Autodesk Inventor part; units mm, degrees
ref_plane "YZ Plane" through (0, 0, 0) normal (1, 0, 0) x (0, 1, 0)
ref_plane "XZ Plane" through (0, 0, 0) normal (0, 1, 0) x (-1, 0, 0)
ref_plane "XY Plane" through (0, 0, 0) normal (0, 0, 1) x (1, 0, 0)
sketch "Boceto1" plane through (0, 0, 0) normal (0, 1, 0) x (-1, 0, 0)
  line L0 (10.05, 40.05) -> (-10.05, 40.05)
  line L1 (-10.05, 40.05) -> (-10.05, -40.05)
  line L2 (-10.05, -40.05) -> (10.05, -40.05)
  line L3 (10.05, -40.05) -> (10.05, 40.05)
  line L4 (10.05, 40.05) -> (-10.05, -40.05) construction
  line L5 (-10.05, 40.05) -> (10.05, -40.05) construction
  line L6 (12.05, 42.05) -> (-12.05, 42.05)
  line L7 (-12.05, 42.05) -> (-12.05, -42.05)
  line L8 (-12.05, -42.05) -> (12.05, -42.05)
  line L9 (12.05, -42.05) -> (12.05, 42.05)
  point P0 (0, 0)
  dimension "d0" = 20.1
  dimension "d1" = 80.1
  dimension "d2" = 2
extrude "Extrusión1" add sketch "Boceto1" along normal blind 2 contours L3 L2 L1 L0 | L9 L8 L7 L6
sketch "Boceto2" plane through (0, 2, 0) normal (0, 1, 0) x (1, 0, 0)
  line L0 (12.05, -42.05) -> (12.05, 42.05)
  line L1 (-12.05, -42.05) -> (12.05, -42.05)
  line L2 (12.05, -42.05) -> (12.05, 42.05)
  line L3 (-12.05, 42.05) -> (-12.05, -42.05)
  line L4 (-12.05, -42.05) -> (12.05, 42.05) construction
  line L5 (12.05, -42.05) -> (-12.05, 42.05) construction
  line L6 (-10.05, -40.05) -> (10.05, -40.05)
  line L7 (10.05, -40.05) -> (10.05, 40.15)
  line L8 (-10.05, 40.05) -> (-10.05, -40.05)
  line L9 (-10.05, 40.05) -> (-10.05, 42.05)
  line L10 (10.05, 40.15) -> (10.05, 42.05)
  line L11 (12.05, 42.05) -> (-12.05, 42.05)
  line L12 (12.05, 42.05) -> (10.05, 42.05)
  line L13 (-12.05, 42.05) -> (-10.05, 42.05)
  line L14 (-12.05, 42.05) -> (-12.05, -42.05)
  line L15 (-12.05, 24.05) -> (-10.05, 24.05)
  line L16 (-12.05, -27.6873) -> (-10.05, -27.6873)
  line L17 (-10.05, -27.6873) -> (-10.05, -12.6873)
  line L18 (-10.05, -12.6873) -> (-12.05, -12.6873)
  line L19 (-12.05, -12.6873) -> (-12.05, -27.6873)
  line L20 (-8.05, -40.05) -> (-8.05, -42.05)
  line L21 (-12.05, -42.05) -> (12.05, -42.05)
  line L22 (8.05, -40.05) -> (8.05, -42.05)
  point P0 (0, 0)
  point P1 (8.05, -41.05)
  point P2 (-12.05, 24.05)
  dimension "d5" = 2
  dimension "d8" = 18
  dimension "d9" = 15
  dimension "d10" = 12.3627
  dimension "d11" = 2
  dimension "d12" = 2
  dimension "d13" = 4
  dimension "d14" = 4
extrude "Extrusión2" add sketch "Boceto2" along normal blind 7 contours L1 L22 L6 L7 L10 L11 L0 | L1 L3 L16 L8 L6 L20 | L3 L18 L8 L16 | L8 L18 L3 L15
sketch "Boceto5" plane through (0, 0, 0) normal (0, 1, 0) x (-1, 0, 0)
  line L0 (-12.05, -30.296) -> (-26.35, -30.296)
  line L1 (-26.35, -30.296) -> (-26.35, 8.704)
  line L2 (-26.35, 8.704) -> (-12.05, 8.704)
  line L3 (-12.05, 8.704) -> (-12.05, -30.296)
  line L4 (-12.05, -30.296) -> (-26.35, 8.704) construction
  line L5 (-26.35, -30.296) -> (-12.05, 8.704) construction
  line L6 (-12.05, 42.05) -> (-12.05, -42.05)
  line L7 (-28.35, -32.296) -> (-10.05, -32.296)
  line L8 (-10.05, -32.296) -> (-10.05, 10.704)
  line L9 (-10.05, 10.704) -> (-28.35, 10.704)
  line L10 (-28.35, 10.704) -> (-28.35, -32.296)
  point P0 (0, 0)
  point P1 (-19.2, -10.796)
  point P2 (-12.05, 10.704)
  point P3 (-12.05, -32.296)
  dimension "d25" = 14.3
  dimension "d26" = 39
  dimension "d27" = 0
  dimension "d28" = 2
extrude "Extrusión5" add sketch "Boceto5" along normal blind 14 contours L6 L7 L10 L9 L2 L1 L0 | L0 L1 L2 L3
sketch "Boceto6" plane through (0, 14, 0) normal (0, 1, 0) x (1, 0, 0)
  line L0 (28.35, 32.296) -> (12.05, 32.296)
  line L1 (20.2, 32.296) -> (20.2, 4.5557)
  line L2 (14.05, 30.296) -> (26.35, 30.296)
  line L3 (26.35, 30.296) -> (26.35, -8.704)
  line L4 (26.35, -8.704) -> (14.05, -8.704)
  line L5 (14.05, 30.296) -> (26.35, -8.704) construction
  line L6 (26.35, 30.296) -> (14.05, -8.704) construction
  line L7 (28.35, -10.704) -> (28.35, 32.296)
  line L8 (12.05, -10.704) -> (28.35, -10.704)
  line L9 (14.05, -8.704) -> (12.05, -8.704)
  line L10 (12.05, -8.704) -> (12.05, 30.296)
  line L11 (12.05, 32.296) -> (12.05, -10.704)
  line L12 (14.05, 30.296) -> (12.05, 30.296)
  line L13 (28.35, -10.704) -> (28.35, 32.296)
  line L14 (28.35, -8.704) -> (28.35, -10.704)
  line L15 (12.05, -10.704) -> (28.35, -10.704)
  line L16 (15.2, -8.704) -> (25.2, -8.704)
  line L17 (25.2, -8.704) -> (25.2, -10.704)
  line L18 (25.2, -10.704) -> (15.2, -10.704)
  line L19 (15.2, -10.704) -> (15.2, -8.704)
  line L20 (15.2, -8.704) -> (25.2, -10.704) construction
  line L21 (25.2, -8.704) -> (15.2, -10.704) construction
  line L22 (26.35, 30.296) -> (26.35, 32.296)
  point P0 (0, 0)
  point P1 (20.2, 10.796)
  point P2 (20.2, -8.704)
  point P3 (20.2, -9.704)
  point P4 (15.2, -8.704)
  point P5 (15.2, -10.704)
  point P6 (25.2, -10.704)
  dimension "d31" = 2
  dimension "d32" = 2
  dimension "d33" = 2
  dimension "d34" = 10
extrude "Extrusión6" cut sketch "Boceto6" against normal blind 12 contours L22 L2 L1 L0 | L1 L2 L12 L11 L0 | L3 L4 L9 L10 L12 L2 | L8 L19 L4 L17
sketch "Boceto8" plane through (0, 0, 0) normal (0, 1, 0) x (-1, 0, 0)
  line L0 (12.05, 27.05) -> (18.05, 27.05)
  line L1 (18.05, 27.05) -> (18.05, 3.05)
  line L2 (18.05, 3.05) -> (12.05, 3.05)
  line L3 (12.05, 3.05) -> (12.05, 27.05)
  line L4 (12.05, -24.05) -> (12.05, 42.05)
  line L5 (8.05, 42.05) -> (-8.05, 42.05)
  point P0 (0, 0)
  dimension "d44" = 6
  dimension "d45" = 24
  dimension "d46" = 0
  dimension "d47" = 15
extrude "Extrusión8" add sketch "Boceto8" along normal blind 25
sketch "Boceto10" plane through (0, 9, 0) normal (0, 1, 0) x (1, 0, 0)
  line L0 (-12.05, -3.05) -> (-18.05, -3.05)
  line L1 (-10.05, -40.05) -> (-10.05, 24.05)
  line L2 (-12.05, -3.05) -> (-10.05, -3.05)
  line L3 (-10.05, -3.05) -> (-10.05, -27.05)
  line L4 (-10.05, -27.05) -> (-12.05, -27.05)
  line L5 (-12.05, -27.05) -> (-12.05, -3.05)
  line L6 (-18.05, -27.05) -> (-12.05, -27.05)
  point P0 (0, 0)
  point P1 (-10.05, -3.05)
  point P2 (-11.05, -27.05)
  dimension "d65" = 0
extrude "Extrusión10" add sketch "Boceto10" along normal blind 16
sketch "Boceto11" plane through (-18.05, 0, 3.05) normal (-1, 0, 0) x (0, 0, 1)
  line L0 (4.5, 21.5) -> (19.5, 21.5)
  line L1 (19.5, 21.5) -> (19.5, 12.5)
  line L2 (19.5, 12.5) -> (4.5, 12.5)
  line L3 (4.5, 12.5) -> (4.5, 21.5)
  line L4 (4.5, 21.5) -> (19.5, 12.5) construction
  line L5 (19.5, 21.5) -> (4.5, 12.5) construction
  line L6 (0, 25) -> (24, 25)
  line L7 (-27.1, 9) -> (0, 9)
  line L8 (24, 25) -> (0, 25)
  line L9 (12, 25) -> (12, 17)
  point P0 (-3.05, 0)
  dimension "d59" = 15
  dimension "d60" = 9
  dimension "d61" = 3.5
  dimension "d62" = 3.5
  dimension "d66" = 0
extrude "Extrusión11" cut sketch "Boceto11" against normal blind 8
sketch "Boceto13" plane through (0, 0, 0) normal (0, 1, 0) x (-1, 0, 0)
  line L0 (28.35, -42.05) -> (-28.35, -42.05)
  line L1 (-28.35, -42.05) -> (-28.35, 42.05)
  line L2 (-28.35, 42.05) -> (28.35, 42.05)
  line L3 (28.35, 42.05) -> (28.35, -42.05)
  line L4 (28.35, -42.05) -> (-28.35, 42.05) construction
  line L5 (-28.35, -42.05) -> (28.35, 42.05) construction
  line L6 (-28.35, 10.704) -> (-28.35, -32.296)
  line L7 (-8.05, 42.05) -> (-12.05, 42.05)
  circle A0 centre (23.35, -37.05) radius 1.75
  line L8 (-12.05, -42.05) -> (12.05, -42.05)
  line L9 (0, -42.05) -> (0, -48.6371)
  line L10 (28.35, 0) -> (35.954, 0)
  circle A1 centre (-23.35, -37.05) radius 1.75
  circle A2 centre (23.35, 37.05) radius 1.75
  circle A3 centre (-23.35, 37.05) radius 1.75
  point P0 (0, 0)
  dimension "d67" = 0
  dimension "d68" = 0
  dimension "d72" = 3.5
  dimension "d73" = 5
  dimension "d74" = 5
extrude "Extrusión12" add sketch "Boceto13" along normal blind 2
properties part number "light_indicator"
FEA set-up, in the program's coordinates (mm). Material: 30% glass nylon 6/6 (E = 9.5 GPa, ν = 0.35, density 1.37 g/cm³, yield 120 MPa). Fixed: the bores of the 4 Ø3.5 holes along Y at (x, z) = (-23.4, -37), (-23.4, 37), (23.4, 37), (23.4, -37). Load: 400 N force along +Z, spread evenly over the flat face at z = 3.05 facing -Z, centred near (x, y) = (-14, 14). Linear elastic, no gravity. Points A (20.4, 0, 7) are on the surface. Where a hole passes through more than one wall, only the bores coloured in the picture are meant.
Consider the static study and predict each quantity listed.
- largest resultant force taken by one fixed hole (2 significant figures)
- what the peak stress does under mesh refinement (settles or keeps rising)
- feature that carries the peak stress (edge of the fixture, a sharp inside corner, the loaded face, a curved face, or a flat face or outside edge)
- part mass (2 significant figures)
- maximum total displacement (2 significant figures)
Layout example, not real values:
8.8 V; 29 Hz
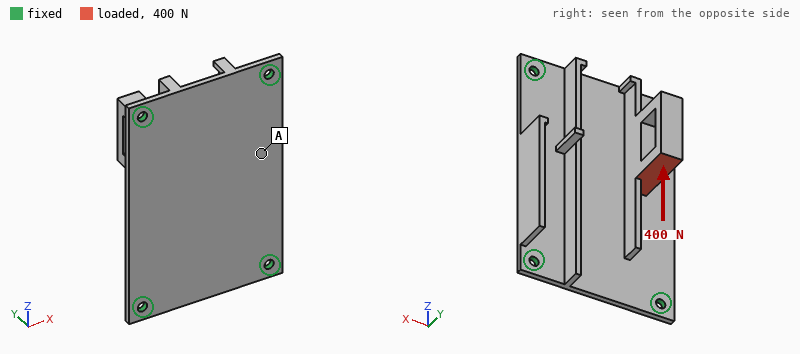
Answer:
160 N; keeps rising; edge of the fixture; 22 g; 0.48 mm
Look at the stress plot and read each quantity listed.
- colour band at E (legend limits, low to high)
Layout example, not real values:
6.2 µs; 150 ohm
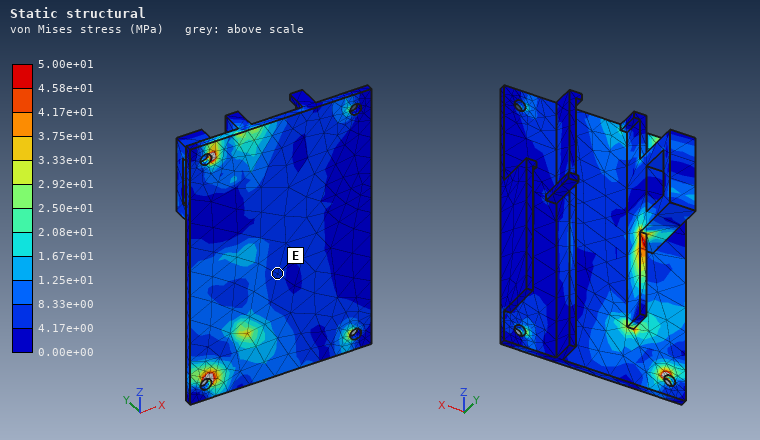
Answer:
4.17e+00 to 8.33e+00 MPa
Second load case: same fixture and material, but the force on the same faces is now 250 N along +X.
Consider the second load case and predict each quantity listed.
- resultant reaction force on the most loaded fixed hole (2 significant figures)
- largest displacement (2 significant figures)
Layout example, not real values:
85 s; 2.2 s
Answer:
130 N; 1.2 mm
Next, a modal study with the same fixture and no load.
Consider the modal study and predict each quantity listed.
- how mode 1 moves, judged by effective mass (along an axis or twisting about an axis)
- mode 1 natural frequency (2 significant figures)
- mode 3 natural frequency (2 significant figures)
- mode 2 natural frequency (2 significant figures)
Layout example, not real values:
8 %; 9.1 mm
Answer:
along Y; 1100 Hz; 1500 Hz; 1300 Hz
